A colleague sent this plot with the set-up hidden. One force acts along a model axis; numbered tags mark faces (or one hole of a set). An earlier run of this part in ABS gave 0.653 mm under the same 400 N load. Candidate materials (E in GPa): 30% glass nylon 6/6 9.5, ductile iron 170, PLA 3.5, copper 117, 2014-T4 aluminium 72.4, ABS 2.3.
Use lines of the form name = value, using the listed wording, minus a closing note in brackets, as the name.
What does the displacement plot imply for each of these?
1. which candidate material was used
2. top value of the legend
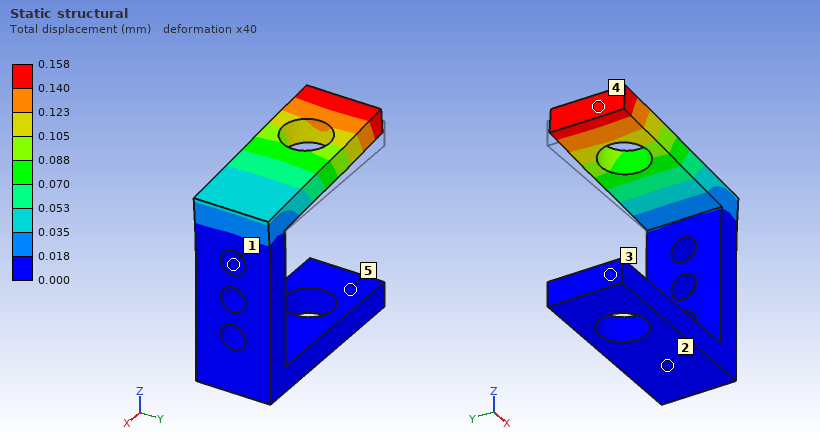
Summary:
which candidate material was used = 30% glass nylon 6/6
top value of the legend = 0.158 mm
